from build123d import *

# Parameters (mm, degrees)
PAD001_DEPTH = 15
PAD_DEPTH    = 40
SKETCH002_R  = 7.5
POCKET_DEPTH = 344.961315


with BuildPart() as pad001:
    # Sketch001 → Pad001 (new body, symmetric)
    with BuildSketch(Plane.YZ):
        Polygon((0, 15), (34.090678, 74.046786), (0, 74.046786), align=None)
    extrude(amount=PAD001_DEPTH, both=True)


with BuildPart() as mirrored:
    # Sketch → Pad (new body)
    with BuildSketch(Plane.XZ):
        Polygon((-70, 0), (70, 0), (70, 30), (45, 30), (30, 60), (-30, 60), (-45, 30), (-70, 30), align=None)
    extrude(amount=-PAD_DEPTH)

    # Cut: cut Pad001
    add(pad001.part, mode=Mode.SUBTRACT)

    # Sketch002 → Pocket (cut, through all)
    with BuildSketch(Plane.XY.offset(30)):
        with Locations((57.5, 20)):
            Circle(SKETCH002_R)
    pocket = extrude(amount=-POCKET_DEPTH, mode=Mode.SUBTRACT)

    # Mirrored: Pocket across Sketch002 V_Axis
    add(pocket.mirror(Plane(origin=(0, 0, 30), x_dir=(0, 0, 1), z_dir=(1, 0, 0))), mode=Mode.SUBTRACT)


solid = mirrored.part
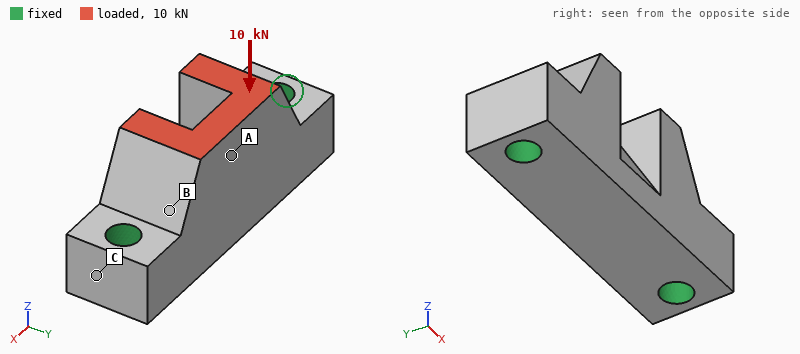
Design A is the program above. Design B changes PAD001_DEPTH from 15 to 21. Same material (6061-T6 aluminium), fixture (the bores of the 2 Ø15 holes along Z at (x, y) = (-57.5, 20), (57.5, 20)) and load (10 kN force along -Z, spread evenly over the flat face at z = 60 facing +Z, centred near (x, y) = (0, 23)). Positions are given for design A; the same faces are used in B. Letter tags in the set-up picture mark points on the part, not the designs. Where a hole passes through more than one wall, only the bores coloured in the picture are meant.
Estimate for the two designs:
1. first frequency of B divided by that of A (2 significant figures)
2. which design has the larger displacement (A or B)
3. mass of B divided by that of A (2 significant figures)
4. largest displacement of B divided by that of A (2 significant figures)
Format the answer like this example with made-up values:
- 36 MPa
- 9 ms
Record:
- 1.0
- B
- 0.97
- 1.2
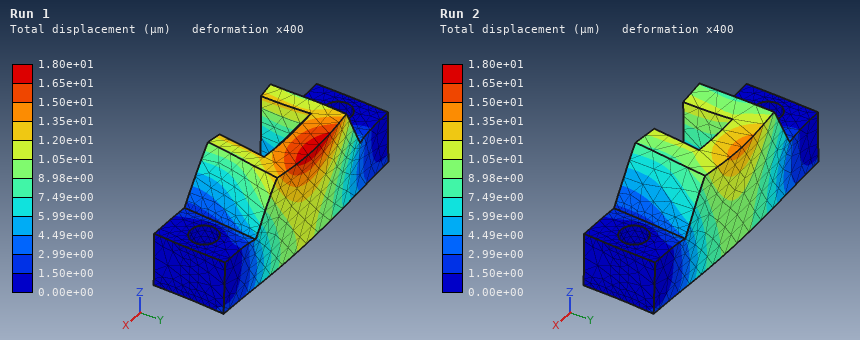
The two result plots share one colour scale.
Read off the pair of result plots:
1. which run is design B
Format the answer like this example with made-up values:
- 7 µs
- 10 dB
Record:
- Run 1
